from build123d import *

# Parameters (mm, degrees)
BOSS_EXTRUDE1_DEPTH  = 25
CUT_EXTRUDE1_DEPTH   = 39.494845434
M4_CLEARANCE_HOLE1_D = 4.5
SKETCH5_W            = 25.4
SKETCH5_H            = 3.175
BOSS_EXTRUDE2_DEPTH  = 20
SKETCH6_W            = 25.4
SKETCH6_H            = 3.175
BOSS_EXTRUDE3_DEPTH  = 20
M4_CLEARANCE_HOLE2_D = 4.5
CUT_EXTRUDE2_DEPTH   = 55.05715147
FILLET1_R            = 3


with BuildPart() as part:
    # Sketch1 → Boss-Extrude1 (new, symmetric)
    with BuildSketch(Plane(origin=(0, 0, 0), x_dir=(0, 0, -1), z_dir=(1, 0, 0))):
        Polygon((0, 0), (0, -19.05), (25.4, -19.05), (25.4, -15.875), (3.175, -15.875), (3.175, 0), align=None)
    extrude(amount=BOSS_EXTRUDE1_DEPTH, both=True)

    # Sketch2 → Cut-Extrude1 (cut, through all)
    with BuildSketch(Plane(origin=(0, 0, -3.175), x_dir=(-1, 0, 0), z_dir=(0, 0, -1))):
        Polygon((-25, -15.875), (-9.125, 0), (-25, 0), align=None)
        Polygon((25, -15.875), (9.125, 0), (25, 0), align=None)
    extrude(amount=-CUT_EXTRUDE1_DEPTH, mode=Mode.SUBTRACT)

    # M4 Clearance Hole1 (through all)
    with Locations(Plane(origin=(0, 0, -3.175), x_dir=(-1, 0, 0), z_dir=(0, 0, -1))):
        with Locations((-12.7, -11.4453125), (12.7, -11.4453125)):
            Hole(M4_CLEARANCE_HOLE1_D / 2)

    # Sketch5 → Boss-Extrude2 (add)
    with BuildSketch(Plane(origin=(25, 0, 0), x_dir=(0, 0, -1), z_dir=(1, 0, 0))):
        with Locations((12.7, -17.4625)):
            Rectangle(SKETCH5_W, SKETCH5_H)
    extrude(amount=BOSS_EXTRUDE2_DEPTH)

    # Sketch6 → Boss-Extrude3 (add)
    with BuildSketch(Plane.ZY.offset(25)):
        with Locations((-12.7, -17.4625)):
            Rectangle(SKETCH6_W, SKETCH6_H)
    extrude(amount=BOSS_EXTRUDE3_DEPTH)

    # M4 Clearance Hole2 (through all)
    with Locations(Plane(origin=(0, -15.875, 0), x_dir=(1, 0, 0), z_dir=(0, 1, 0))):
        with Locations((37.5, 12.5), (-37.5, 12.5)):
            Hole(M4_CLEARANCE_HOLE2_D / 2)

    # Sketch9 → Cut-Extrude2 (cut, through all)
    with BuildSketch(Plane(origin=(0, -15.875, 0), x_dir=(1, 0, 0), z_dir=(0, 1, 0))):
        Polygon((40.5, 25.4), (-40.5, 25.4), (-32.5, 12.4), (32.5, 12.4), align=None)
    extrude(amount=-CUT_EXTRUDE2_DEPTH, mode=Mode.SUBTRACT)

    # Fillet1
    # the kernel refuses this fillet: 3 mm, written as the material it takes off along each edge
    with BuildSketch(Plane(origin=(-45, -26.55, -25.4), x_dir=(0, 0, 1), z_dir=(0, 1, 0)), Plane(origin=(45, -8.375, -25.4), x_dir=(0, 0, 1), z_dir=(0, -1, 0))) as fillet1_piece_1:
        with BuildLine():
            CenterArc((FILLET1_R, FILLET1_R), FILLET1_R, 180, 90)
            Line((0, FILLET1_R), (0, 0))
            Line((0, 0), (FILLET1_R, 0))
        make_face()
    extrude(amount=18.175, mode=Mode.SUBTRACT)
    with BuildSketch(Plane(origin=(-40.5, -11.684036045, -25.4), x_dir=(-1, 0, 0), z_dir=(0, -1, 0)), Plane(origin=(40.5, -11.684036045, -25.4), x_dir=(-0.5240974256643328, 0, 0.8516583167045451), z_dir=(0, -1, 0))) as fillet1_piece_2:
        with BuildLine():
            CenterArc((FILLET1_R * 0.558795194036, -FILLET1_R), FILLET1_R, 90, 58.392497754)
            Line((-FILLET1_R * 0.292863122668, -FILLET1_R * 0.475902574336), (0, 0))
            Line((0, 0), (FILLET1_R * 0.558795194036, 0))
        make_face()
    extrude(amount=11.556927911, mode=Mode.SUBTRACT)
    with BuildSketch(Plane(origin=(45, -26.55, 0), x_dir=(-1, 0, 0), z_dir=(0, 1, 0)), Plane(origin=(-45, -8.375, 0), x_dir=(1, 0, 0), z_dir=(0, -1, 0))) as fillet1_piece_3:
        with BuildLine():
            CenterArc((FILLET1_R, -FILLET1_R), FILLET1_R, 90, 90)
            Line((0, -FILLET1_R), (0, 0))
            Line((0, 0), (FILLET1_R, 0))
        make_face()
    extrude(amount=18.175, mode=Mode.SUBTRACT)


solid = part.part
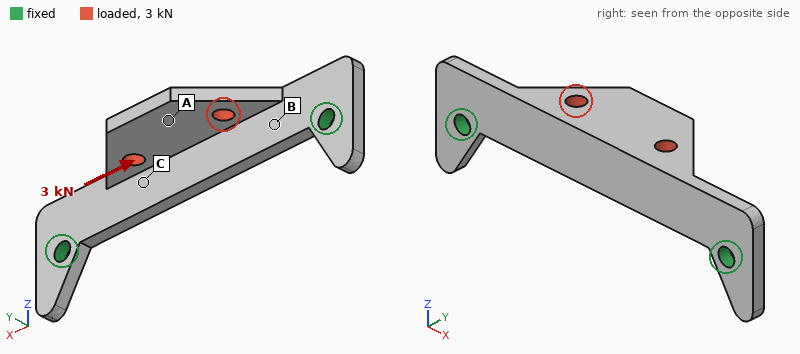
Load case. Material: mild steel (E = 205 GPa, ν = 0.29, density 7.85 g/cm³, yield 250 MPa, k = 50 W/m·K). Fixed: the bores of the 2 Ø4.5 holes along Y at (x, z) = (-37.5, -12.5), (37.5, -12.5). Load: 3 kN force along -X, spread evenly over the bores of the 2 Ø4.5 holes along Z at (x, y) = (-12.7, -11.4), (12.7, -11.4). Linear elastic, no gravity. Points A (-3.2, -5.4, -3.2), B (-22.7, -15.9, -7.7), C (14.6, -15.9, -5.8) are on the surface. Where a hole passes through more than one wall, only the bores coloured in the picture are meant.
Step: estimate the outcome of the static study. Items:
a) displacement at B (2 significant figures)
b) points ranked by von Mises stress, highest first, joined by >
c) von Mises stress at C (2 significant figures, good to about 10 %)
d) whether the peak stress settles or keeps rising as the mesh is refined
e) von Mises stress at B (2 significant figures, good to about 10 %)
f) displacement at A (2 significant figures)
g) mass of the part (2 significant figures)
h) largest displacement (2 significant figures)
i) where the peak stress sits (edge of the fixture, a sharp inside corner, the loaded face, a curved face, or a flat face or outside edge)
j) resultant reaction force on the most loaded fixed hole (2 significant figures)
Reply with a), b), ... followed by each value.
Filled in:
a) 15 µm
b) B > C > A
c) 58 MPa
d) keeps rising
e) 96 MPa
f) 21 µm
g) 45 g
h) 29 µm
i) edge of the fixture
j) 1.6 kN
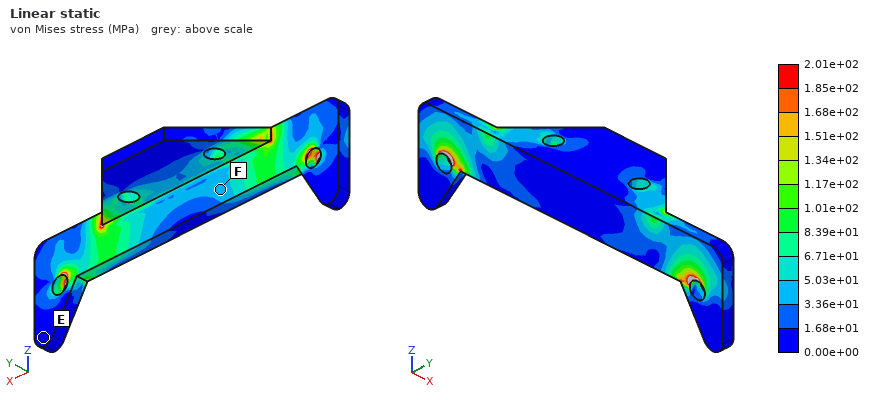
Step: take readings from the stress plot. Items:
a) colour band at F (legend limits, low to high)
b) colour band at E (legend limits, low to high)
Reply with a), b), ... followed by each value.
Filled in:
a) 3.36e+01 to 5.03e+01 MPa
b) 0.00e+00 to 1.68e+01 MPa
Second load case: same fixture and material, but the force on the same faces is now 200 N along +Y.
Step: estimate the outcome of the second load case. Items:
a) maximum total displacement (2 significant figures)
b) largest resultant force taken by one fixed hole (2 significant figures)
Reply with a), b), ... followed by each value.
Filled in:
a) 27 µm
b) 100 N
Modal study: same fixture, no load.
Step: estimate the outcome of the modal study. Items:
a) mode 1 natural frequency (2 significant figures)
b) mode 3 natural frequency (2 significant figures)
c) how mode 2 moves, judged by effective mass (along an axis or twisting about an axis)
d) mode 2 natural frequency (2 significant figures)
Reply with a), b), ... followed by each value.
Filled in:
a) 3100 Hz
b) 8000 Hz
c) along Y
d) 4300 Hz
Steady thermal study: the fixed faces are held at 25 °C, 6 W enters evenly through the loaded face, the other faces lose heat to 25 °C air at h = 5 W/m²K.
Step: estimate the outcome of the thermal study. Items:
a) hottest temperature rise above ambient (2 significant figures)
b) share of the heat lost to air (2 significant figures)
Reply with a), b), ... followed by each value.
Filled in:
a) 41 K
b) 8.0 %
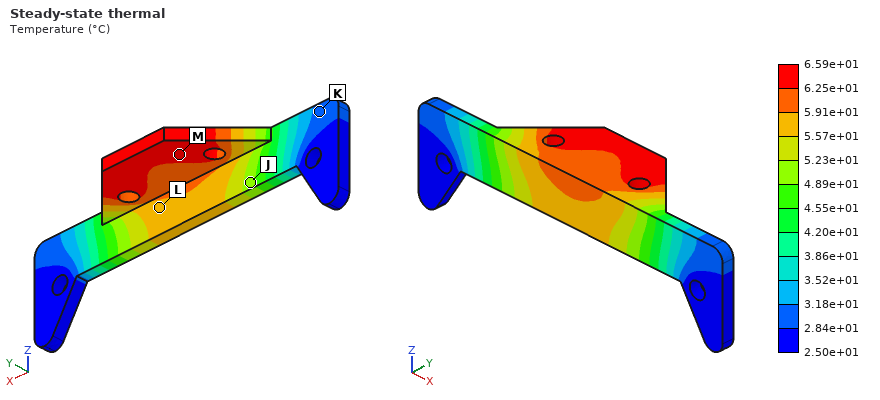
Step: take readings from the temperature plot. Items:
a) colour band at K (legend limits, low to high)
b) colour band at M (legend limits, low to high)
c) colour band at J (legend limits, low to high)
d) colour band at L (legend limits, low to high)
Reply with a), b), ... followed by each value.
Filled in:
a) 2.84e+01 to 3.18e+01 °C
b) 6.25e+01 to 6.59e+01 °C
c) 4.89e+01 to 5.23e+01 °C
d) 5.57e+01 to 5.91e+01 °C
